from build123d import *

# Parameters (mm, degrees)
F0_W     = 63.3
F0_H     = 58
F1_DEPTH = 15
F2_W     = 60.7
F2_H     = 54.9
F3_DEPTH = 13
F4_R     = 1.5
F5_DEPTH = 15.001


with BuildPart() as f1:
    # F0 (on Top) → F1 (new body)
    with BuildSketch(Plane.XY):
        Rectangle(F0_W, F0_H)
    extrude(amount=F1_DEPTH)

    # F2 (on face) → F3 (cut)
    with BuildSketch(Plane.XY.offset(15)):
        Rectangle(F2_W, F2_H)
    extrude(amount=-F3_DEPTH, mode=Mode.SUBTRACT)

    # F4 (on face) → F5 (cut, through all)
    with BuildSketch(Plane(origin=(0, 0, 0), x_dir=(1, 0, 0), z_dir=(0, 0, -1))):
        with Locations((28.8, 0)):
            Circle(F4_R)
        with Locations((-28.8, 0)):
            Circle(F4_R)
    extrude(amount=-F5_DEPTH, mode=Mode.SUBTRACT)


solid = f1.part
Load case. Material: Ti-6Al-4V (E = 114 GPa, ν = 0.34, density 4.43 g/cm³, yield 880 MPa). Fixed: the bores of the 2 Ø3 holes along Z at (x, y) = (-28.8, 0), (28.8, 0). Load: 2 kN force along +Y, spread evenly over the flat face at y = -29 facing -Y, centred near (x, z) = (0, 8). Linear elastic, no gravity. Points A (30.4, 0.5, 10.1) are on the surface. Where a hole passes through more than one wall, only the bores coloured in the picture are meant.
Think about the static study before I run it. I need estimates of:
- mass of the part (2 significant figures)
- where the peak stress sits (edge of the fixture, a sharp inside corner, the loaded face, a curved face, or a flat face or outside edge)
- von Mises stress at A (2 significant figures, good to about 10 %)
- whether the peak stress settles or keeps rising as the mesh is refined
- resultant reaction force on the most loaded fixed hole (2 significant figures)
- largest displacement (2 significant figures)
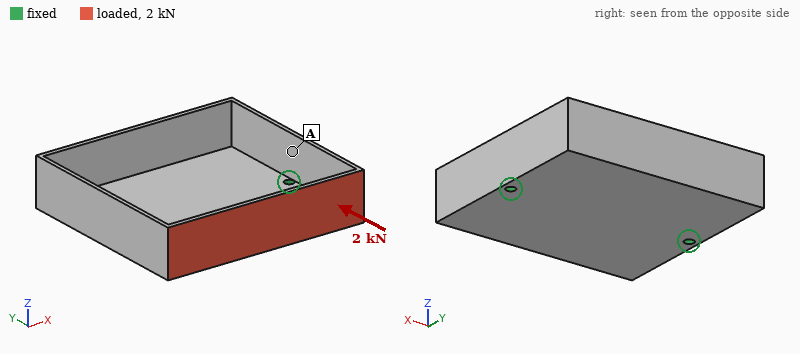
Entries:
52 g
edge of the fixture
44 MPa
keeps rising
1.0 kN
0.57 mm
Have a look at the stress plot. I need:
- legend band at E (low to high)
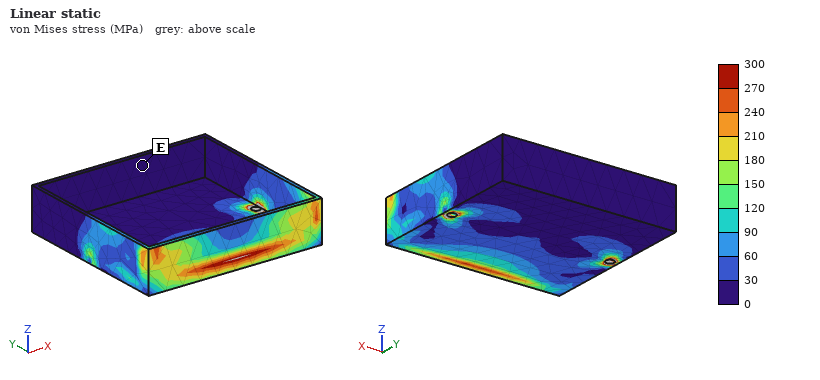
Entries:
0 to 30 MPa
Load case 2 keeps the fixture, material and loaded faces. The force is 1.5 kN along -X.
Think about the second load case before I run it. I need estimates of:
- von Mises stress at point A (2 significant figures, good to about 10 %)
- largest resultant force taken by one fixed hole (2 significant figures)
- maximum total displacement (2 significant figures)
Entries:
46 MPa
1.1 kN
0.16 mm
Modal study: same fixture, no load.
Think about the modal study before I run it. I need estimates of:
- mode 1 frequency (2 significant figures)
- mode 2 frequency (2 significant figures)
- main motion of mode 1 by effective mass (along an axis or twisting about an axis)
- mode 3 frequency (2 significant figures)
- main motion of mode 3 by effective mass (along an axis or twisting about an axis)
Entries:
1500 Hz
2400 Hz
twisting about X
3600 Hz
along Z
